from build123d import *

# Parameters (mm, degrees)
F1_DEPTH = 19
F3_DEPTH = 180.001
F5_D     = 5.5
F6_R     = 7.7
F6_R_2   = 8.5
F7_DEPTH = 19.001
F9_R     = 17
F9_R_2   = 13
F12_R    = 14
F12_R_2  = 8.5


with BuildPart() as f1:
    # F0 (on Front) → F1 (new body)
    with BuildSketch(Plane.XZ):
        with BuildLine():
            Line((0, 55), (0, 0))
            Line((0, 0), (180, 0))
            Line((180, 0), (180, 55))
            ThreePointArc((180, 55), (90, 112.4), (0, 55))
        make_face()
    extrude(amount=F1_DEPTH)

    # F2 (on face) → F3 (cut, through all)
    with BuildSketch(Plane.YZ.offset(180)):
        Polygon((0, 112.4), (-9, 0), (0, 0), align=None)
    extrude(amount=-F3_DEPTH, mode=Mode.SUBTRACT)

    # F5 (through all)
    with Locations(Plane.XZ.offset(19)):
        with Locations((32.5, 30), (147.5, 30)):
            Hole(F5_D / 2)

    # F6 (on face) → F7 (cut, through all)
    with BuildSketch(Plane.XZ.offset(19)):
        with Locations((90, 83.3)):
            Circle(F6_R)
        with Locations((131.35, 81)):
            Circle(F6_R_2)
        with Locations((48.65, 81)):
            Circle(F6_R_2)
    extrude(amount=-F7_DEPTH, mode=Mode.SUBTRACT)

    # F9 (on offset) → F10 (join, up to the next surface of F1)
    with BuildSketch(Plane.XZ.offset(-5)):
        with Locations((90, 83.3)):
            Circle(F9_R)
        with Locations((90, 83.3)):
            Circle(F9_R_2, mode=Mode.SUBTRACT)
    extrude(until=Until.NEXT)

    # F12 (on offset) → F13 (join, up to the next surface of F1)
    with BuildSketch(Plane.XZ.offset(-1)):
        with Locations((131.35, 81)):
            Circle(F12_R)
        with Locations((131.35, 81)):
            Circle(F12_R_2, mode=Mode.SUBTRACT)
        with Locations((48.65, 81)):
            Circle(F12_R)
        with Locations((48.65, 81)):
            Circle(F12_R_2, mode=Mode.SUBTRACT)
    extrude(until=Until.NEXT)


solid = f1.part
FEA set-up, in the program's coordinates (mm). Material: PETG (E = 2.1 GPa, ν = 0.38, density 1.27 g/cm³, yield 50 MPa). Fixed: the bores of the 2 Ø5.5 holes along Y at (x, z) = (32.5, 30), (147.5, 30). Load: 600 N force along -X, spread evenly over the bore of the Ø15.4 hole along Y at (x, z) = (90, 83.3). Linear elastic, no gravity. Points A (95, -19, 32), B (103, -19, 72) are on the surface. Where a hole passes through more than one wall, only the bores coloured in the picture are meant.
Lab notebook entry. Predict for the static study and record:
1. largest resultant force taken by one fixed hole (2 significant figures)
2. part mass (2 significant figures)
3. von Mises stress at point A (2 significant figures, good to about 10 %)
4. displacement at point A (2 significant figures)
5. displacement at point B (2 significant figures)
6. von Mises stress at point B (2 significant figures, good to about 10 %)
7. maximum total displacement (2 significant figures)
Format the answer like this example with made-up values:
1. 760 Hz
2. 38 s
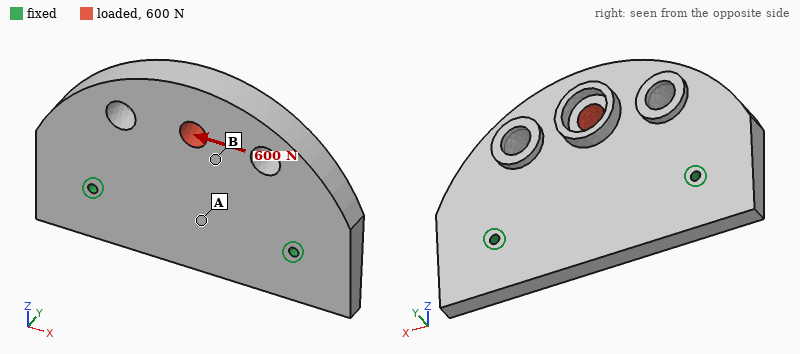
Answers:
1. 410 N
2. 300 g
3. 0.29 MPa
4. 9.6 µm
5. 30 µm
6. 0.76 MPa
7. 44 µm
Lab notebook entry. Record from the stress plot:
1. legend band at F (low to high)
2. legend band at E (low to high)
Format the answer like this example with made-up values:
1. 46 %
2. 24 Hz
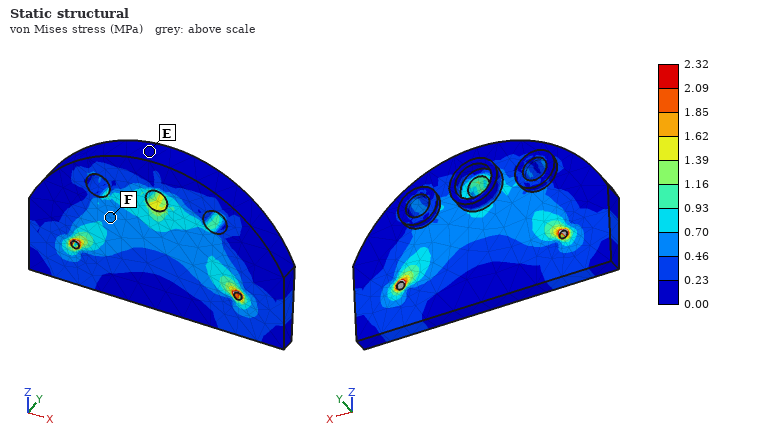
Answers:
1. 0.46 to 0.70 MPa
2. 0.00 to 0.23 MPa
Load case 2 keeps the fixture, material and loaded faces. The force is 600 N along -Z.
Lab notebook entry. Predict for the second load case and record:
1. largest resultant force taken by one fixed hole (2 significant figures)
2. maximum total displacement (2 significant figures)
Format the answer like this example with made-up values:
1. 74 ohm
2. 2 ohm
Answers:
1. 320 N
2. 86 µm
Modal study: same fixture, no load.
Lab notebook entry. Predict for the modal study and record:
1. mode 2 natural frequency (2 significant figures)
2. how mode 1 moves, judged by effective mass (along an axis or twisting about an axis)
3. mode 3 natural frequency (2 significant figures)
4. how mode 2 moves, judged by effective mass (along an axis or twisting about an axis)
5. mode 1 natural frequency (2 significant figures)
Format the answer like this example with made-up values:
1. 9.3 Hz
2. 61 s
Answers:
1. 800 Hz
2. along Y
3. 930 Hz
4. twisting about Z
5. 310 Hz
